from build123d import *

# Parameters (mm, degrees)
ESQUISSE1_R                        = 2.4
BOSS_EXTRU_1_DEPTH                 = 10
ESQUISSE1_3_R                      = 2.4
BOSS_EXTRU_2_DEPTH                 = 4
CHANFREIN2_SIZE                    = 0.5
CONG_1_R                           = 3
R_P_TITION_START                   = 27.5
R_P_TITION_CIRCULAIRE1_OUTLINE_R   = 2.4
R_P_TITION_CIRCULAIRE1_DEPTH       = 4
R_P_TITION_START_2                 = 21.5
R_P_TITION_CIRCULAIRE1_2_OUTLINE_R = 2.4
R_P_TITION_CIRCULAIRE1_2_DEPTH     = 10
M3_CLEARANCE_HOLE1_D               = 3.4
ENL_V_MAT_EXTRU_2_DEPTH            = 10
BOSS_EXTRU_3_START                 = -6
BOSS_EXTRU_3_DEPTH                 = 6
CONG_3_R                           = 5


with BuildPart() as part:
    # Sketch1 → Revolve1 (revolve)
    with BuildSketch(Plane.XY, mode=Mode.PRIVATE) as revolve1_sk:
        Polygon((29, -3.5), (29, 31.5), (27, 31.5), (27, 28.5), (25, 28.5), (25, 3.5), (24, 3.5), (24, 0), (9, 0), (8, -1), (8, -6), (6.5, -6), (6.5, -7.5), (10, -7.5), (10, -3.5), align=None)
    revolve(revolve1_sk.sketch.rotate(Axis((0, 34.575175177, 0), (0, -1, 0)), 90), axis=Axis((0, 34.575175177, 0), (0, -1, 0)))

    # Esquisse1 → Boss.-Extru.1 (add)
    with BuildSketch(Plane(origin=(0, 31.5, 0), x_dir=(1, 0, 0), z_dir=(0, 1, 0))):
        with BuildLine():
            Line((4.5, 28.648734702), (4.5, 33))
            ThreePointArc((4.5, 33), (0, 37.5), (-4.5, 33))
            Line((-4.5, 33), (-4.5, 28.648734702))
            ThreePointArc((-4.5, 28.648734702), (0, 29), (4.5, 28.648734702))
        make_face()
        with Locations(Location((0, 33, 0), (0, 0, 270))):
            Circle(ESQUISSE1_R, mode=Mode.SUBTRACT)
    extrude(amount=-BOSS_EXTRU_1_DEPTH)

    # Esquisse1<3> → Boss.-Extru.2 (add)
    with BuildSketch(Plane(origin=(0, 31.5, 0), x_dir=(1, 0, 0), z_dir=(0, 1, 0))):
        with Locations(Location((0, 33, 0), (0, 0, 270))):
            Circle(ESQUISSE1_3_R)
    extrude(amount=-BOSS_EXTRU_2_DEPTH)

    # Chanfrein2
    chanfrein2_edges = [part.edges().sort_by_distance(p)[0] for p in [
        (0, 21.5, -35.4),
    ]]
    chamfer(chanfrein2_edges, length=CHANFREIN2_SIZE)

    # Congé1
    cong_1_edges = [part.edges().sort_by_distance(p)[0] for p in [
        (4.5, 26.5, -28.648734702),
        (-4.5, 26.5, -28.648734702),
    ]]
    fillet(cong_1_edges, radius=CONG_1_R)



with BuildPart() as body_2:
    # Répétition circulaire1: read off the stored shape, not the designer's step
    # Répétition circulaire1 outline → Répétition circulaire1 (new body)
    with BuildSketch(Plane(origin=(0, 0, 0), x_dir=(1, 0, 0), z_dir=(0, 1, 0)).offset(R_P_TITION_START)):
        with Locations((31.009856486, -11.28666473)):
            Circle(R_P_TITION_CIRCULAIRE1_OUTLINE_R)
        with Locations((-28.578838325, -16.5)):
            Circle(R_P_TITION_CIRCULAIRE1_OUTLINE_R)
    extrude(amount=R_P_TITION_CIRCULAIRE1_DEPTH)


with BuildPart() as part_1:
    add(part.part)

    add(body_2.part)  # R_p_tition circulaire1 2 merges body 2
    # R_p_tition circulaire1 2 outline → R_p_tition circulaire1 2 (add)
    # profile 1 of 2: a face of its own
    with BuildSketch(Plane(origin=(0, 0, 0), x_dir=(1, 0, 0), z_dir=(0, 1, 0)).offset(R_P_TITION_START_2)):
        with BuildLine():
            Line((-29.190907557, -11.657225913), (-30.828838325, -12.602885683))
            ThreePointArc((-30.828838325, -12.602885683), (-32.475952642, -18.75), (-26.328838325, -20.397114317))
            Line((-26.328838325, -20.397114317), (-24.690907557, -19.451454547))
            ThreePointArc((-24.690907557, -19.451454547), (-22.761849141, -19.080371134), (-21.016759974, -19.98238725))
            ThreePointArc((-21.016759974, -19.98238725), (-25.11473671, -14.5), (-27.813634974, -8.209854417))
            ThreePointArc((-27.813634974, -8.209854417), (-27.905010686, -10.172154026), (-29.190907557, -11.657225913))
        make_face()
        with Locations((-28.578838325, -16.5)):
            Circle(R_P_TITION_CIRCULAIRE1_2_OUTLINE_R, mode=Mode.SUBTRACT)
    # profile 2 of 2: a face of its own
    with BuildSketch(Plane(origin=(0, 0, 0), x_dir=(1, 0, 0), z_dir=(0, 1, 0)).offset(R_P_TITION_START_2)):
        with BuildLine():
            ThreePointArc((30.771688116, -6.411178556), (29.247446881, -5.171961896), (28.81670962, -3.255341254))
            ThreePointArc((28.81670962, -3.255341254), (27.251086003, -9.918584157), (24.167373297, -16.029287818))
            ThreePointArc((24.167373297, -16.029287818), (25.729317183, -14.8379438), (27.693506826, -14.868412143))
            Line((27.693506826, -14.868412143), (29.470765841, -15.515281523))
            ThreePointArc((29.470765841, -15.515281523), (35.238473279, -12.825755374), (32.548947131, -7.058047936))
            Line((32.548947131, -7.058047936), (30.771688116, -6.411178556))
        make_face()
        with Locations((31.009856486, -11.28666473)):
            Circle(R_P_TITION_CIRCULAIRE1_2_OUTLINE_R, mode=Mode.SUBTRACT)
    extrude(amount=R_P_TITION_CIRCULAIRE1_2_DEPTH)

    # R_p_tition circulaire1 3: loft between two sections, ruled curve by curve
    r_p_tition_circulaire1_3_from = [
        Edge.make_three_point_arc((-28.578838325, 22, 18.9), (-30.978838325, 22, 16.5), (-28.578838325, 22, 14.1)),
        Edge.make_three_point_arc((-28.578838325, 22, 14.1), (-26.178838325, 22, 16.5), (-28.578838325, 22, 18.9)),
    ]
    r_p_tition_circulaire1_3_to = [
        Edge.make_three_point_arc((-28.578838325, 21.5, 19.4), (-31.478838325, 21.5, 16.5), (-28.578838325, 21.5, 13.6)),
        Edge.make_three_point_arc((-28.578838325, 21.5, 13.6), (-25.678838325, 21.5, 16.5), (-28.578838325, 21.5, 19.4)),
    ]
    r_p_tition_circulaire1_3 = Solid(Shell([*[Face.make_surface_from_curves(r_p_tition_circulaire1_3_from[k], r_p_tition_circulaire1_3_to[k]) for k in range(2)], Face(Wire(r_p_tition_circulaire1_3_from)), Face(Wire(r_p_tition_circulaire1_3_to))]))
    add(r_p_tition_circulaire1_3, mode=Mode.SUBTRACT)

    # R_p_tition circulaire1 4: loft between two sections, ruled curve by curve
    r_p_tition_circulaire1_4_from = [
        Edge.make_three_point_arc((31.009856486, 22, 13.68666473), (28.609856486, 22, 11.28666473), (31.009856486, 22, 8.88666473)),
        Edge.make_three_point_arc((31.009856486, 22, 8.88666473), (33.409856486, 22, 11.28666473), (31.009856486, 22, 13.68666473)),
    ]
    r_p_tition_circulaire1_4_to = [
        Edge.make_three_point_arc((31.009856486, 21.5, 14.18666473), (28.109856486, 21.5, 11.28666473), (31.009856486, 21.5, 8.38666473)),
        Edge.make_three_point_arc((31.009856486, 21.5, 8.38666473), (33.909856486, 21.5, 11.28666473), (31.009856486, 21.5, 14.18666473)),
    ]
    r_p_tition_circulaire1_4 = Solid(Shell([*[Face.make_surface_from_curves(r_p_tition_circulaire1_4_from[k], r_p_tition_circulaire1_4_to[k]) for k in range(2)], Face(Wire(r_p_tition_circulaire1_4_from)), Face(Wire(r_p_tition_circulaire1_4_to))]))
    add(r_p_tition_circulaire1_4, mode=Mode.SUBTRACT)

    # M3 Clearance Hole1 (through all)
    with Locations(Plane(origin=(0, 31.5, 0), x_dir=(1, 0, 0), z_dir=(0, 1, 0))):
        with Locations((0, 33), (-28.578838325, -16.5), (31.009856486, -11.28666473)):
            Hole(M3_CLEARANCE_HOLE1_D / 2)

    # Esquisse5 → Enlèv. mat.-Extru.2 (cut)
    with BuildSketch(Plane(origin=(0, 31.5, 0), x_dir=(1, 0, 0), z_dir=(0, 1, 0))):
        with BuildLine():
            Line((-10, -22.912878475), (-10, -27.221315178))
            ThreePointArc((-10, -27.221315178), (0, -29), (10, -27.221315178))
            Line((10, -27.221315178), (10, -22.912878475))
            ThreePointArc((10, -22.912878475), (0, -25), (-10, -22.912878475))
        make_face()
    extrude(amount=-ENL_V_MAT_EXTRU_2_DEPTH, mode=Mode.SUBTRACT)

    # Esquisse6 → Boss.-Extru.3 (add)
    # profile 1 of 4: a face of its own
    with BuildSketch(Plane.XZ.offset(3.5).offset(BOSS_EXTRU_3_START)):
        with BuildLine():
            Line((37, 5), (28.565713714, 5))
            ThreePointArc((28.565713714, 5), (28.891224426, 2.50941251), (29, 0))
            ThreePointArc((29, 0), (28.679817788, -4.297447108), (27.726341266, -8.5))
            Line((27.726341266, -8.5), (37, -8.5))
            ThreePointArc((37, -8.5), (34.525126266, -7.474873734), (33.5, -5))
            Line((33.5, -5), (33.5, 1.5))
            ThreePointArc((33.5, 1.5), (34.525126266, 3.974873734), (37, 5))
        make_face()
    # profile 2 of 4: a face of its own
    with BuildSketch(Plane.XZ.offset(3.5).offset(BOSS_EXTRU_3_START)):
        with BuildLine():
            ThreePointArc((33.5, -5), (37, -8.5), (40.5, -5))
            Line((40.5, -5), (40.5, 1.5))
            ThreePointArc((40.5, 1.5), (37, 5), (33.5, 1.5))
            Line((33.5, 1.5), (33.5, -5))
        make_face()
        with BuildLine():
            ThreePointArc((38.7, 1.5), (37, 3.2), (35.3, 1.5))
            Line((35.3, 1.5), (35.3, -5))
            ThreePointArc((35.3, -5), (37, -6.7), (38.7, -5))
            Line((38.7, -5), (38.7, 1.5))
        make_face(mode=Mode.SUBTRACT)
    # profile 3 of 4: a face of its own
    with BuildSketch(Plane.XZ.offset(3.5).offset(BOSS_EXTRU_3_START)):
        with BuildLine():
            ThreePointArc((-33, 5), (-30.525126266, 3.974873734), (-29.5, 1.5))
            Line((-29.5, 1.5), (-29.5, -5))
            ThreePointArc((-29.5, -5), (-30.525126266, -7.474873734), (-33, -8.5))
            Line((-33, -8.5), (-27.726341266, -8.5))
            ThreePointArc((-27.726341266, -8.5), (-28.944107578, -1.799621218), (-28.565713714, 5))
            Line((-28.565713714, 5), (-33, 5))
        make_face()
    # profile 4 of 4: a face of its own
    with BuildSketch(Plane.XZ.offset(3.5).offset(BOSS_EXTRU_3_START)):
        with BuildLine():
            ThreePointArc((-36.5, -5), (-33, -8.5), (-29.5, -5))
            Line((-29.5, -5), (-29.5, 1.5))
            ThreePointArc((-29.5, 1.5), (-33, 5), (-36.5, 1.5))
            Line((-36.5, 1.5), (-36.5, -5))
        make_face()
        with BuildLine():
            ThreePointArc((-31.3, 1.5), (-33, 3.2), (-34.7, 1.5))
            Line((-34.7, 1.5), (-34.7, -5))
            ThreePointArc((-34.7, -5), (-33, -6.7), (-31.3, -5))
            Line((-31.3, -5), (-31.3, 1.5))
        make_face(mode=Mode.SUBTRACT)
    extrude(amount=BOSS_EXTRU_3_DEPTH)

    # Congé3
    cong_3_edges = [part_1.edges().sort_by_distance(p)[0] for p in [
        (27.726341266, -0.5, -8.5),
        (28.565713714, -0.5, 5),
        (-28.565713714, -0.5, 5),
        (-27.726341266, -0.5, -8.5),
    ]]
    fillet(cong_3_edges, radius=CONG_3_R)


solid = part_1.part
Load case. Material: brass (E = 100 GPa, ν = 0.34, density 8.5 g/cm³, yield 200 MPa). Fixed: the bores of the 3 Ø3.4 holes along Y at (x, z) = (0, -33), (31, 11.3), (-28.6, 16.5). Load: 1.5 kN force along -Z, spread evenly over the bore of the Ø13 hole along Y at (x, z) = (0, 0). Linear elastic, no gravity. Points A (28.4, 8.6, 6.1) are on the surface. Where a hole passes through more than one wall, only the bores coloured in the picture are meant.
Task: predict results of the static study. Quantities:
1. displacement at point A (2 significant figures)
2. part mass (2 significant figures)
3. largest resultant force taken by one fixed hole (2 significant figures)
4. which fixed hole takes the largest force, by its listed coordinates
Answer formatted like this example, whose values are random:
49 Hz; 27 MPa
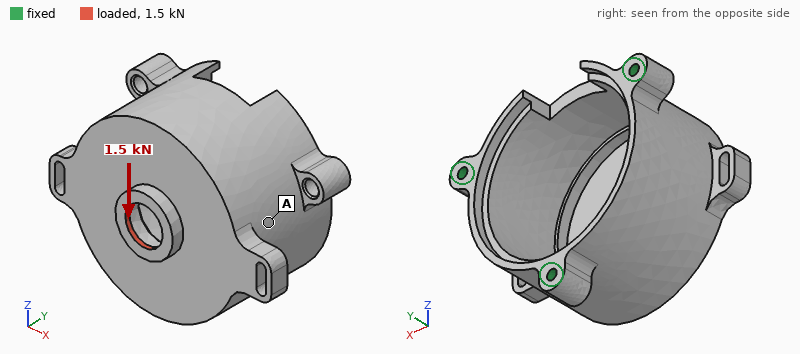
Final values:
8.6 µm; 270 g; 1.3 kN; (0, -33)
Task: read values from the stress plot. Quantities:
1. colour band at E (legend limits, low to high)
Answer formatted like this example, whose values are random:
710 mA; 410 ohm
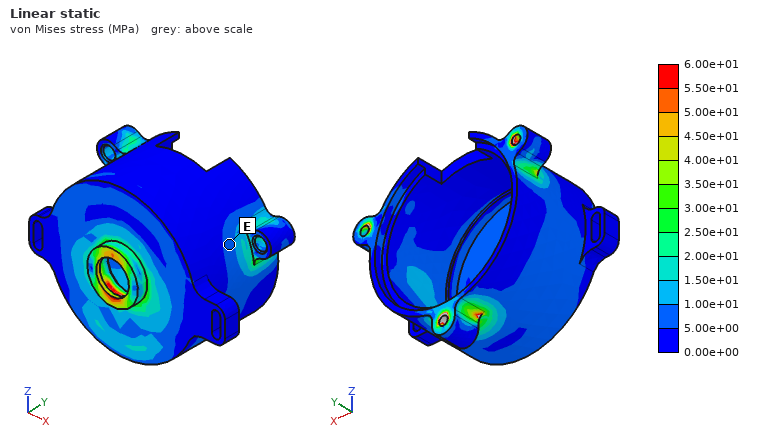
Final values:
5.00e+00 to 1.00e+01 MPa
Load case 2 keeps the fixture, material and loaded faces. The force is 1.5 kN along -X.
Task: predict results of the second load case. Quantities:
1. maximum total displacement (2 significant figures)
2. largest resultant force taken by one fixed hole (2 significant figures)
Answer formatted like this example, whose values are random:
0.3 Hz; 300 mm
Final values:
23 µm; 1.1 kN
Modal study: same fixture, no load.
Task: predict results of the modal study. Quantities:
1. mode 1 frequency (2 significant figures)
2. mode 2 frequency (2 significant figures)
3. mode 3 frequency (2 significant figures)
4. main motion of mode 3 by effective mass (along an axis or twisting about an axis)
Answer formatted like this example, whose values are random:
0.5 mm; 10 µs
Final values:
4200 Hz; 4500 Hz; 6300 Hz; along Y
